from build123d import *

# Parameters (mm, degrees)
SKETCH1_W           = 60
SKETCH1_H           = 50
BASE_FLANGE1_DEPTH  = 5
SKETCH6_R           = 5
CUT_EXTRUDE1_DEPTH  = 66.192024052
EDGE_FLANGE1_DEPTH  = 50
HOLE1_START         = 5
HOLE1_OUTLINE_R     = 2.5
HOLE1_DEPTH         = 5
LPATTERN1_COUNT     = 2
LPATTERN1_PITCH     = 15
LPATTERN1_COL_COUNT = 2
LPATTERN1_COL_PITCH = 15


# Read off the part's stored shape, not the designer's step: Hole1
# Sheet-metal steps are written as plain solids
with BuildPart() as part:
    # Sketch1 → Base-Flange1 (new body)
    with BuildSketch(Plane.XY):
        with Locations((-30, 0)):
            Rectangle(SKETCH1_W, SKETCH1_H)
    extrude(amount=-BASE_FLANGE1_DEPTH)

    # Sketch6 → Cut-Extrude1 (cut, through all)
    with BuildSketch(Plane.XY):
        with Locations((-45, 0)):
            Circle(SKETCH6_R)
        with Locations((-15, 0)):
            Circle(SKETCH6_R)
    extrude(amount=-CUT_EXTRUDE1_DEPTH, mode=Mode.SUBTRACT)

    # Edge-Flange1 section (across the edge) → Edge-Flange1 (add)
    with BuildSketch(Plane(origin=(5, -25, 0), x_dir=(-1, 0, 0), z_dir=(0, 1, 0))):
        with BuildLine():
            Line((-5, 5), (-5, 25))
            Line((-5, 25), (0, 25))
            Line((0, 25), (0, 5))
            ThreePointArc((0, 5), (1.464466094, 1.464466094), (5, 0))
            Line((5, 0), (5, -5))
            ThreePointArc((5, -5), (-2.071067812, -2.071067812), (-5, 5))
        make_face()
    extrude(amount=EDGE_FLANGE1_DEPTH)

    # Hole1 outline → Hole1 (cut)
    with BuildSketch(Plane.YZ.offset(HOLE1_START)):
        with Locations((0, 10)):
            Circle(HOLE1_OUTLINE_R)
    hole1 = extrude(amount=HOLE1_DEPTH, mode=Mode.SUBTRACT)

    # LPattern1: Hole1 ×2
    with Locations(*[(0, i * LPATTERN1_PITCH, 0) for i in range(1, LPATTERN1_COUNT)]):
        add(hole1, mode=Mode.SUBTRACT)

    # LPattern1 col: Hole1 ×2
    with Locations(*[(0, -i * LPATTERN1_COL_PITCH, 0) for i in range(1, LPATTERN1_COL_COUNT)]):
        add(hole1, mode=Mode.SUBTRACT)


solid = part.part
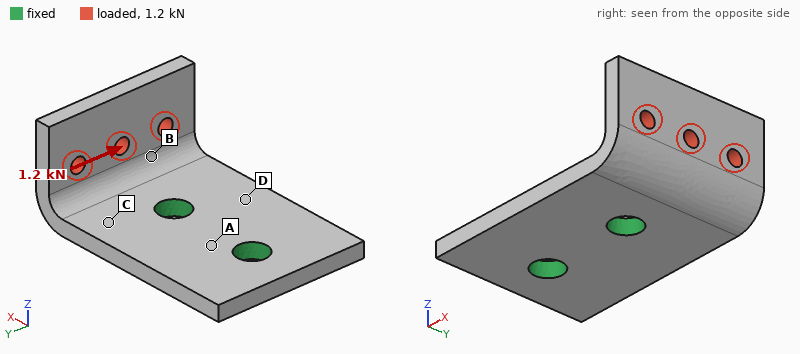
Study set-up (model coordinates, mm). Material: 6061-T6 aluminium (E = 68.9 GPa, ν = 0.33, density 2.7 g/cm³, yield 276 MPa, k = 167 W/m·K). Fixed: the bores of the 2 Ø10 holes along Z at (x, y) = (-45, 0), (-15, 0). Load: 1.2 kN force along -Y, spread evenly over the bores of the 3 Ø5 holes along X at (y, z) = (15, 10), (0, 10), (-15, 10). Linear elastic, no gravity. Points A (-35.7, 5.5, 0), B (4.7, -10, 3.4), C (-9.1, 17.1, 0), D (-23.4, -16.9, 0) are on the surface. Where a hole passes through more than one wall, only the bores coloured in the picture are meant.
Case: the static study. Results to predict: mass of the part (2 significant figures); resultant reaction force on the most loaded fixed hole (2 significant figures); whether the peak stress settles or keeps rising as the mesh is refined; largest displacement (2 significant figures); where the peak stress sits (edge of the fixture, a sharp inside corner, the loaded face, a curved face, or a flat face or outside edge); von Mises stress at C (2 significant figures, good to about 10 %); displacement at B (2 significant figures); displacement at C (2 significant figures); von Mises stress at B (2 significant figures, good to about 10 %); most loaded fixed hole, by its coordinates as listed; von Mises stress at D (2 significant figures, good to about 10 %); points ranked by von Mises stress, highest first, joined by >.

59 g
1.7 kN
keeps rising
0.17 mm
edge of the fixture
30 MPa
0.050 mm
0.033 mm
44 MPa
(-15, 0)
18 MPa
B > C > D > A
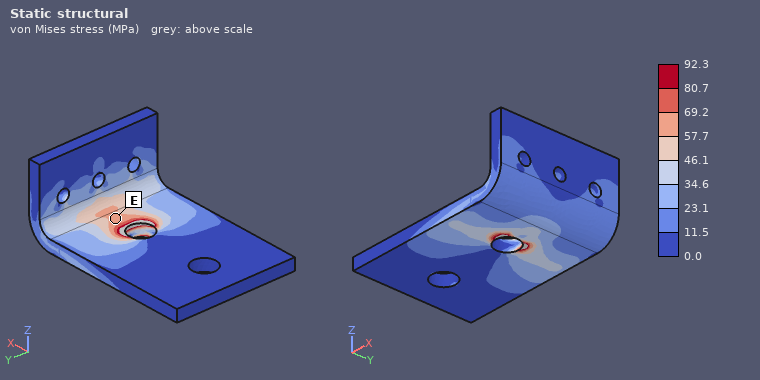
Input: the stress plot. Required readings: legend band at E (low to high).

57.7 to 69.2 MPa
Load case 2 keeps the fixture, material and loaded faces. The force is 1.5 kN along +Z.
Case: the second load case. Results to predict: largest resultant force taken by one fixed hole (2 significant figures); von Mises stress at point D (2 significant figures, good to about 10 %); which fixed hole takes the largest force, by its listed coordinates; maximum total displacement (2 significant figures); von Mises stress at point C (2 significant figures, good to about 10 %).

1.7 kN
23 MPa
(-15, 0)
0.30 mm
67 MPa
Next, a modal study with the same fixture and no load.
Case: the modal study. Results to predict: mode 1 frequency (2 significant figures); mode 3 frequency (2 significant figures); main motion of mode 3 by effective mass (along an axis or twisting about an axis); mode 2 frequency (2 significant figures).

2400 Hz
6600 Hz
along Z
3000 Hz
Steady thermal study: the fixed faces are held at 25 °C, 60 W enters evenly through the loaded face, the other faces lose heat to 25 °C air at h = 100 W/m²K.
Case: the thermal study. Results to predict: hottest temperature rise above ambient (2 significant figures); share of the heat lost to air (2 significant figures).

43 K
25 %
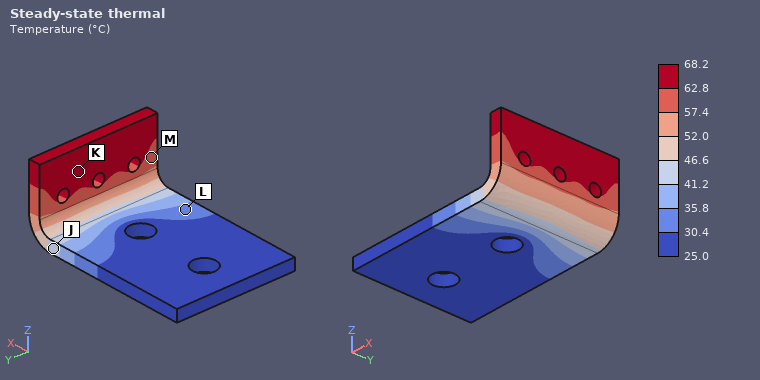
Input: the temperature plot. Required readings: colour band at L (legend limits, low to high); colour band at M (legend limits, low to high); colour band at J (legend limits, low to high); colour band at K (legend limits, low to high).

30.4 to 35.8 °C
57.4 to 62.8 °C
41.2 to 46.6 °C
62.8 to 68.2 °C
